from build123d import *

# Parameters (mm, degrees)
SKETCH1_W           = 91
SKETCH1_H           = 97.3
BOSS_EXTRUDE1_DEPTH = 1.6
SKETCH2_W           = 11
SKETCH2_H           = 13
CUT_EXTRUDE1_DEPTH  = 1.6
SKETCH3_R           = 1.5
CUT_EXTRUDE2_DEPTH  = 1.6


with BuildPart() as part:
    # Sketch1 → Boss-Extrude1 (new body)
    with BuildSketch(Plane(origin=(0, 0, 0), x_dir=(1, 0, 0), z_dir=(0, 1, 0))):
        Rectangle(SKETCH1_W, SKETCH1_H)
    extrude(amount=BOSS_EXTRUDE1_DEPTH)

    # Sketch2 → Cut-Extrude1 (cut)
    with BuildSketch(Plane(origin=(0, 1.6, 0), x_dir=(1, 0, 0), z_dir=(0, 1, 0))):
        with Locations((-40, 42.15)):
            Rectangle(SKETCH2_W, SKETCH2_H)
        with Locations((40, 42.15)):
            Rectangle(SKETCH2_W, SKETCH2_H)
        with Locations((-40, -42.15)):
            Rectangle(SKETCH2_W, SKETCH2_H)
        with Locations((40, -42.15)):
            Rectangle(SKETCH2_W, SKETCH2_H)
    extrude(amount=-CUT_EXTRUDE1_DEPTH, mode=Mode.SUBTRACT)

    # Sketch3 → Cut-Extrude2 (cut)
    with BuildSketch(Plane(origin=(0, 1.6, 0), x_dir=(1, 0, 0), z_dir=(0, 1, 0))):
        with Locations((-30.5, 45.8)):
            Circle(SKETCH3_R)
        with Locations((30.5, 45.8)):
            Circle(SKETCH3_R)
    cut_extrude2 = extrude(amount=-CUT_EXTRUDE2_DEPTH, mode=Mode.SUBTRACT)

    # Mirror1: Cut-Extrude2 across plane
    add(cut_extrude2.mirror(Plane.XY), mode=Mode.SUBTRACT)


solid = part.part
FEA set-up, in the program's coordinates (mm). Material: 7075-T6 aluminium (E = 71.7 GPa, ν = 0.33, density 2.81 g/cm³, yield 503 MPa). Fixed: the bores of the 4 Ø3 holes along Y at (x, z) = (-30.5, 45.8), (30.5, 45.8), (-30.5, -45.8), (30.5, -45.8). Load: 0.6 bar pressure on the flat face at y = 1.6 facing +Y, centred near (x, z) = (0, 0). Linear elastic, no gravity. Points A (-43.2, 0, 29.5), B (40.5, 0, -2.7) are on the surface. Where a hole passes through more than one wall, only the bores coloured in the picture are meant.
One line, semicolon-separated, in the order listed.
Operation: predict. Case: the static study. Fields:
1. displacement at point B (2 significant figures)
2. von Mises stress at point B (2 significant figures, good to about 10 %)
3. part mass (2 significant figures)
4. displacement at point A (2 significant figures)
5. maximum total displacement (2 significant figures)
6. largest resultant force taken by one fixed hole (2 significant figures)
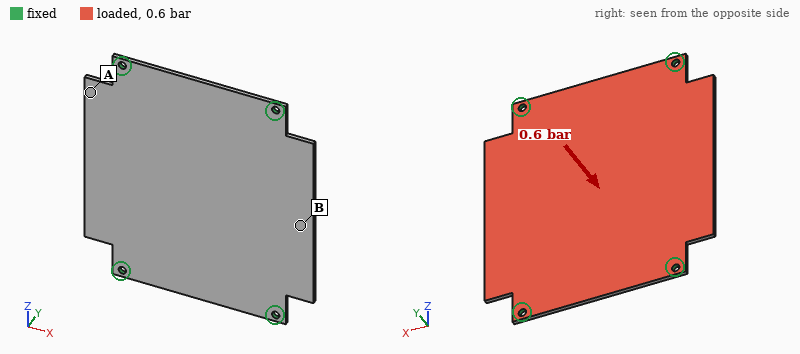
0.76 mm; 71 MPa; 37 g; 0.30 mm; 0.78 mm; 120 N
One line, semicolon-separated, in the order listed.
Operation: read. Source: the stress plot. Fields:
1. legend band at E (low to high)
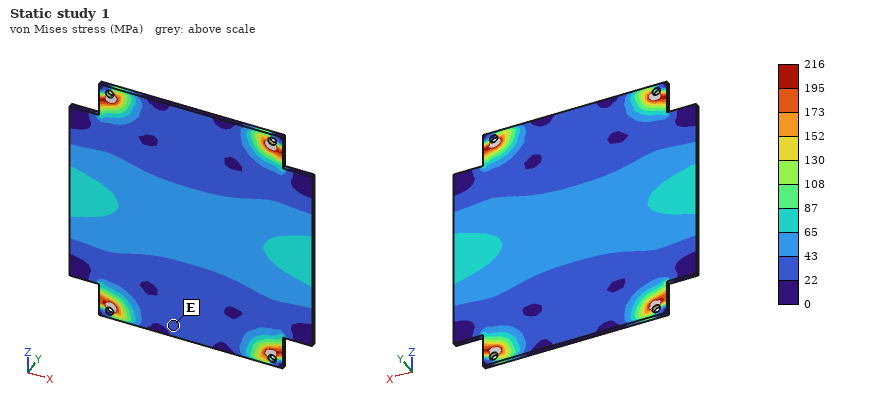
22 to 43 MPa
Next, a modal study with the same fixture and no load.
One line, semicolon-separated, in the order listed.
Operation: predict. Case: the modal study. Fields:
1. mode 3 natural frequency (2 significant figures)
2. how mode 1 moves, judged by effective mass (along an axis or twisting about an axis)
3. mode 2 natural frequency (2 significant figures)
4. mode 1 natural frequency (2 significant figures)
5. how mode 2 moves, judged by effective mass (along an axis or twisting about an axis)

1400 Hz; along Y; 970 Hz; 750 Hz; twisting about Z
